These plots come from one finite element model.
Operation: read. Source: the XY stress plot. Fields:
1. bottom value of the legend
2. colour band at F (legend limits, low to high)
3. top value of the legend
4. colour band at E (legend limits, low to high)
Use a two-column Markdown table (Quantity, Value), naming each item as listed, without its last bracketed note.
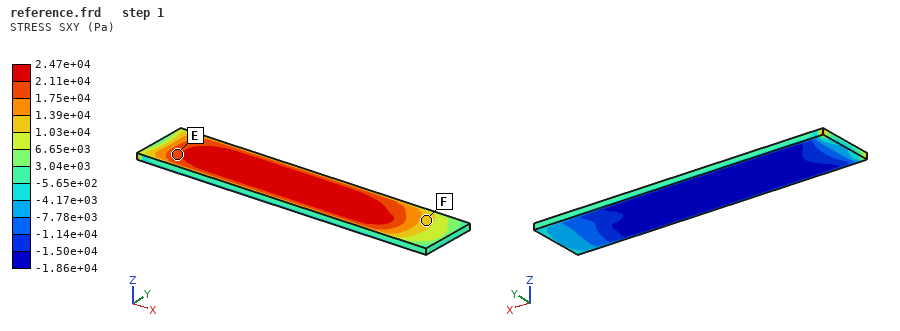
| Quantity | Value |
|---|---|
| bottom value of the legend | -1.86e+04 Pa |
| colour band at F | 1.03e+04 to 1.39e+04 Pa |
| top value of the legend | 2.47e+04 Pa |
| colour band at E | 1.75e+04 to 2.11e+04 Pa |
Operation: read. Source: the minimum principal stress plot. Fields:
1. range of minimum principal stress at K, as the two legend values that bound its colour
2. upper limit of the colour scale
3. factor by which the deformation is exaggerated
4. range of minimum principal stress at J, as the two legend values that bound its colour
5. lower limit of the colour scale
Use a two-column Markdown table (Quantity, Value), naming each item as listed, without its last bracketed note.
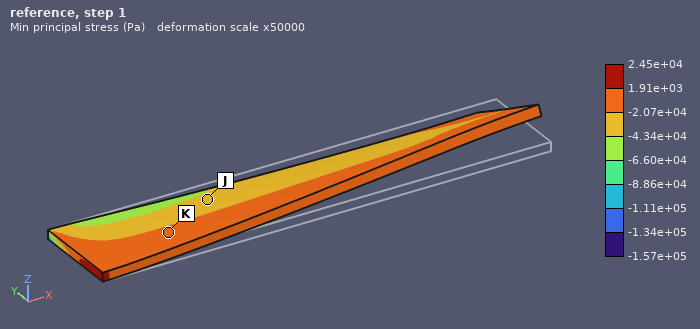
| Quantity | Value |
|---|---|
| range of minimum principal stress at K, as the two legend values that bound its colour | -2.07e+04 to 1.91e+03 Pa |
| upper limit of the colour scale | 2.45e+04 Pa |
| factor by which the deformation is exaggerated | 50000 |
| range of minimum principal stress at J, as the two legend values that bound its colour | -4.34e+04 to -2.07e+04 Pa |
| lower limit of the colour scale | -1.57e+05 Pa |
